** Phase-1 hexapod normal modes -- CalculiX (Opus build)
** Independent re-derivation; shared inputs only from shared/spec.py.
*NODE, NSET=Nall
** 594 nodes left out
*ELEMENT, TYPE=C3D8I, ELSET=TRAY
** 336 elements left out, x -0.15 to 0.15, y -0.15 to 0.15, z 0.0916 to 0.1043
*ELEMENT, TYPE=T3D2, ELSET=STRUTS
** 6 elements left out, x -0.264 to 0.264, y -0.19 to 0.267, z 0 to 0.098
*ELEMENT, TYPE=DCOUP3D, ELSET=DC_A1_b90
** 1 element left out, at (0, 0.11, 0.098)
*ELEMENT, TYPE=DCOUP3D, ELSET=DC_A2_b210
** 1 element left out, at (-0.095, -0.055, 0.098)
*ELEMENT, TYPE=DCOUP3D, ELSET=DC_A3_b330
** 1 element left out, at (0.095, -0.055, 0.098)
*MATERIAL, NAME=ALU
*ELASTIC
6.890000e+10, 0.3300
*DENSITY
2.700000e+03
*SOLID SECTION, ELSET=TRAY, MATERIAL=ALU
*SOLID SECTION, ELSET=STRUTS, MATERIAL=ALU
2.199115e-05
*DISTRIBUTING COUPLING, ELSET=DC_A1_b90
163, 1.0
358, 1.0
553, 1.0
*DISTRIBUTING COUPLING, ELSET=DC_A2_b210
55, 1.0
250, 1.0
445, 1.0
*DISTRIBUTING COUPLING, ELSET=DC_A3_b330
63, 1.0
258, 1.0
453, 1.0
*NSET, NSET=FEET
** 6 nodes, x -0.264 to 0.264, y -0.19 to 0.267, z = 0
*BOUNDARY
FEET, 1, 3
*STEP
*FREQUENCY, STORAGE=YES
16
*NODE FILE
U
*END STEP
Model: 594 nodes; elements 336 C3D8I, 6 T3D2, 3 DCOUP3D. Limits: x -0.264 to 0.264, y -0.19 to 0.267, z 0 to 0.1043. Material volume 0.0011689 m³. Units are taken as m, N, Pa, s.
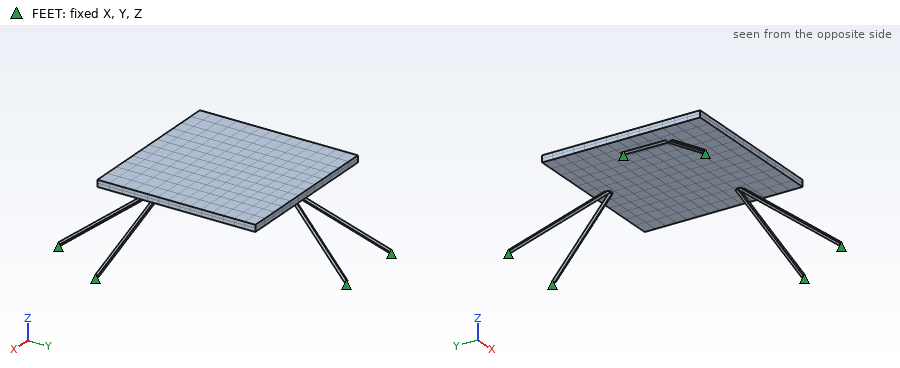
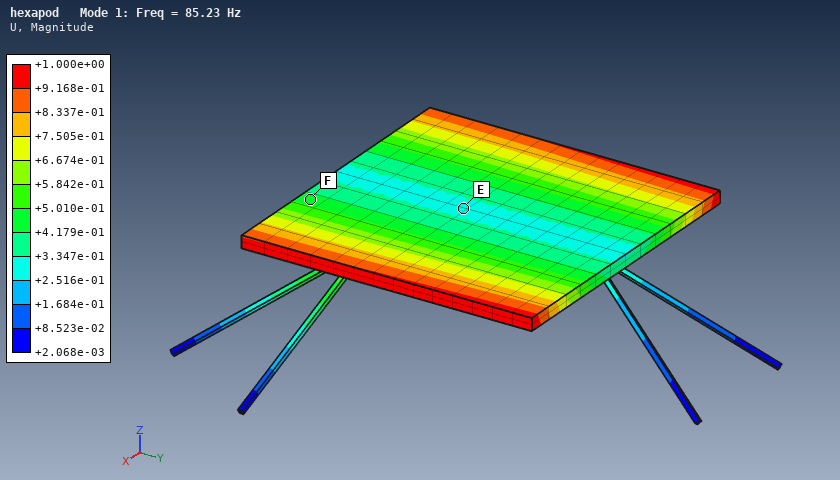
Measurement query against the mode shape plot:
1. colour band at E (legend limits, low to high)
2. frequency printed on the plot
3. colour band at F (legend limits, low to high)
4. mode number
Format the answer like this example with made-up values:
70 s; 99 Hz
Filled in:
+2.516e-01 to +3.347e-01; 85.23 Hz; +4.179e-01 to +5.010e-01; 1
